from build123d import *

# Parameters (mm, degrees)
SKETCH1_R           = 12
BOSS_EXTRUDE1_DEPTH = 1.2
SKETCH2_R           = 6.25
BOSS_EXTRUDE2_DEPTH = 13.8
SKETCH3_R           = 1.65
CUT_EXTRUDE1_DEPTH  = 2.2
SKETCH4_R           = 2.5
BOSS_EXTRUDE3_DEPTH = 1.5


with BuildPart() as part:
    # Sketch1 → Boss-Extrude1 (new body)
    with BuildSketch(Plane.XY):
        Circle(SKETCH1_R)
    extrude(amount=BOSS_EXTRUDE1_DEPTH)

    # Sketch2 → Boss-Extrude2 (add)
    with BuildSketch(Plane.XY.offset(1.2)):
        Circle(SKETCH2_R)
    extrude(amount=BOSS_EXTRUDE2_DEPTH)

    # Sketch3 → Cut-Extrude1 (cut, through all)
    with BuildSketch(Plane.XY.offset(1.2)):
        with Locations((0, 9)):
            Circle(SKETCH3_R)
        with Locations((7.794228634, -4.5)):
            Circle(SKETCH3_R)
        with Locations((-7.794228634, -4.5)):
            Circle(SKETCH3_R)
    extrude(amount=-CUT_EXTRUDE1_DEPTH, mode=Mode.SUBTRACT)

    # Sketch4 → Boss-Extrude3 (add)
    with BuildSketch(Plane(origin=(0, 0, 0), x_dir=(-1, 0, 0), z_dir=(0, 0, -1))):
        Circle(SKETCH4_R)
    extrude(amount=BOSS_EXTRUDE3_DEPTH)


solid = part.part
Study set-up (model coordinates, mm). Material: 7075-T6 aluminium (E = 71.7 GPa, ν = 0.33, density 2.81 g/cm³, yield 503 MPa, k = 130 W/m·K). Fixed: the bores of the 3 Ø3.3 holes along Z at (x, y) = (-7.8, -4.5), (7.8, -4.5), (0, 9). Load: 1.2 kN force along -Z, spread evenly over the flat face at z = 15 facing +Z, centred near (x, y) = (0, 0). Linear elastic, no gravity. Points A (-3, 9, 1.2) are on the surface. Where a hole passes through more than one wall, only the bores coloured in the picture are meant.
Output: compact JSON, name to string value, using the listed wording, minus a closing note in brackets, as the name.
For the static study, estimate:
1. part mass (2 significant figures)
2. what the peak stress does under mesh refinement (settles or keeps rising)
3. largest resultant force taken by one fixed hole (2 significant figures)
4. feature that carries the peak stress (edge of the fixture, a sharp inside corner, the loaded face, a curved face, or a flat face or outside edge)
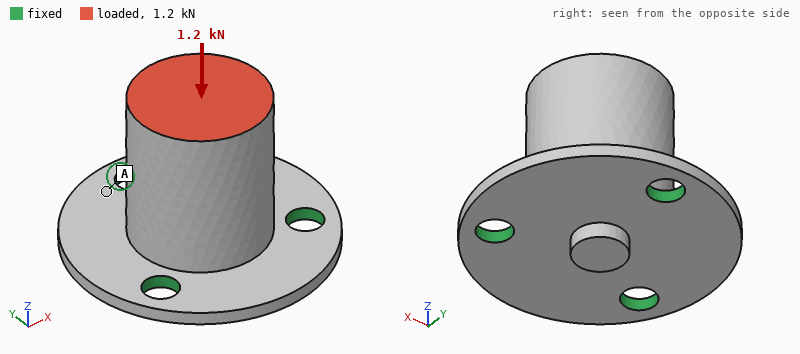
{"part mass": "6.3 g", "what the peak stress does under mesh refinement": "keeps rising", "largest resultant force taken by one fixed hole": "440 N", "feature that carries the peak stress": "edge of the fixture"}
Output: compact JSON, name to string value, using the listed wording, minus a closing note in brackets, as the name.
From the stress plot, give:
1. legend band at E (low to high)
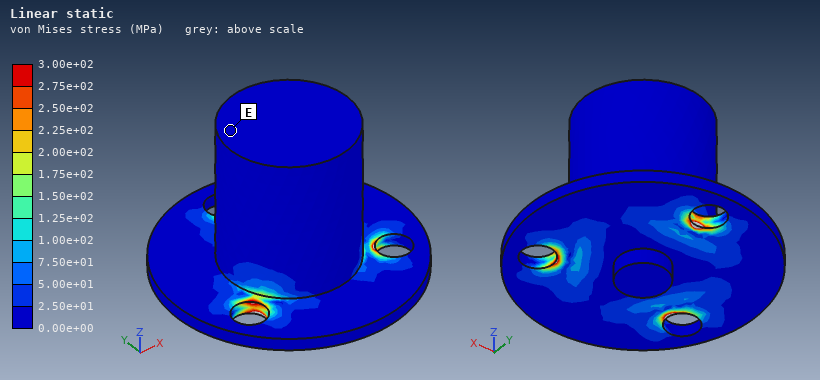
{"legend band at E": "0.00e+00 to 2.50e+01 MPa"}
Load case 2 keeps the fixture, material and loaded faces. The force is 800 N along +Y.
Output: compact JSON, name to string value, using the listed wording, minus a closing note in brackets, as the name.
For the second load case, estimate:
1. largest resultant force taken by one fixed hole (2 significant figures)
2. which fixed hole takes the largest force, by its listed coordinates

{"largest resultant force taken by one fixed hole": "1.1 kN", "which fixed hole takes the largest force, by its listed coordinates": "(0, 9)"}
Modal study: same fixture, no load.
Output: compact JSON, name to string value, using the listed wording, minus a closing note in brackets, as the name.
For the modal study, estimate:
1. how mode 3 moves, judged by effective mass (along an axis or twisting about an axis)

{"how mode 3 moves, judged by effective mass": "along Z"}
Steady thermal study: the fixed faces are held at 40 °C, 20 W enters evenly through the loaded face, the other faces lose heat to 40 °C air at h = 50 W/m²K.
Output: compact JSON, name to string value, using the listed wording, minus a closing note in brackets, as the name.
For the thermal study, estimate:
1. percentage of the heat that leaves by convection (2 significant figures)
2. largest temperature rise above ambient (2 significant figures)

{"percentage of the heat that leaves by convection": "4.6 %", "largest temperature rise above ambient": "31 K"}
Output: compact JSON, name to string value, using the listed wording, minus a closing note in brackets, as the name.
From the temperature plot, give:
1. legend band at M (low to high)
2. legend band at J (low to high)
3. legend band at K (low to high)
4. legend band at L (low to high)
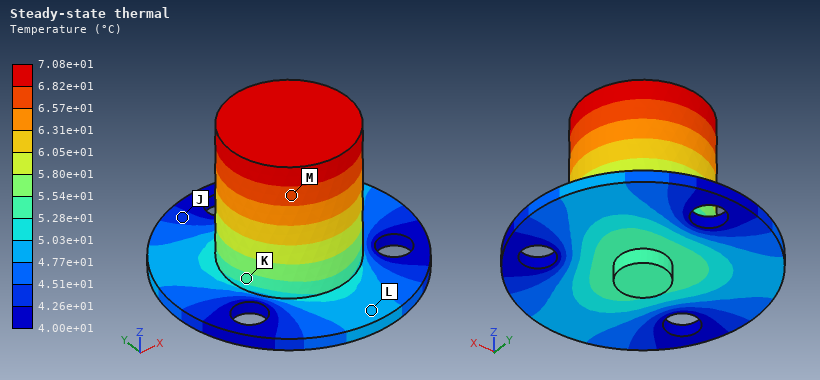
{"legend band at M": "6.57e+01 to 6.82e+01 °C", "legend band at J": "4.26e+01 to 4.51e+01 °C", "legend band at K": "5.28e+01 to 5.54e+01 °C", "legend band at L": "4.77e+01 to 5.03e+01 °C"}
